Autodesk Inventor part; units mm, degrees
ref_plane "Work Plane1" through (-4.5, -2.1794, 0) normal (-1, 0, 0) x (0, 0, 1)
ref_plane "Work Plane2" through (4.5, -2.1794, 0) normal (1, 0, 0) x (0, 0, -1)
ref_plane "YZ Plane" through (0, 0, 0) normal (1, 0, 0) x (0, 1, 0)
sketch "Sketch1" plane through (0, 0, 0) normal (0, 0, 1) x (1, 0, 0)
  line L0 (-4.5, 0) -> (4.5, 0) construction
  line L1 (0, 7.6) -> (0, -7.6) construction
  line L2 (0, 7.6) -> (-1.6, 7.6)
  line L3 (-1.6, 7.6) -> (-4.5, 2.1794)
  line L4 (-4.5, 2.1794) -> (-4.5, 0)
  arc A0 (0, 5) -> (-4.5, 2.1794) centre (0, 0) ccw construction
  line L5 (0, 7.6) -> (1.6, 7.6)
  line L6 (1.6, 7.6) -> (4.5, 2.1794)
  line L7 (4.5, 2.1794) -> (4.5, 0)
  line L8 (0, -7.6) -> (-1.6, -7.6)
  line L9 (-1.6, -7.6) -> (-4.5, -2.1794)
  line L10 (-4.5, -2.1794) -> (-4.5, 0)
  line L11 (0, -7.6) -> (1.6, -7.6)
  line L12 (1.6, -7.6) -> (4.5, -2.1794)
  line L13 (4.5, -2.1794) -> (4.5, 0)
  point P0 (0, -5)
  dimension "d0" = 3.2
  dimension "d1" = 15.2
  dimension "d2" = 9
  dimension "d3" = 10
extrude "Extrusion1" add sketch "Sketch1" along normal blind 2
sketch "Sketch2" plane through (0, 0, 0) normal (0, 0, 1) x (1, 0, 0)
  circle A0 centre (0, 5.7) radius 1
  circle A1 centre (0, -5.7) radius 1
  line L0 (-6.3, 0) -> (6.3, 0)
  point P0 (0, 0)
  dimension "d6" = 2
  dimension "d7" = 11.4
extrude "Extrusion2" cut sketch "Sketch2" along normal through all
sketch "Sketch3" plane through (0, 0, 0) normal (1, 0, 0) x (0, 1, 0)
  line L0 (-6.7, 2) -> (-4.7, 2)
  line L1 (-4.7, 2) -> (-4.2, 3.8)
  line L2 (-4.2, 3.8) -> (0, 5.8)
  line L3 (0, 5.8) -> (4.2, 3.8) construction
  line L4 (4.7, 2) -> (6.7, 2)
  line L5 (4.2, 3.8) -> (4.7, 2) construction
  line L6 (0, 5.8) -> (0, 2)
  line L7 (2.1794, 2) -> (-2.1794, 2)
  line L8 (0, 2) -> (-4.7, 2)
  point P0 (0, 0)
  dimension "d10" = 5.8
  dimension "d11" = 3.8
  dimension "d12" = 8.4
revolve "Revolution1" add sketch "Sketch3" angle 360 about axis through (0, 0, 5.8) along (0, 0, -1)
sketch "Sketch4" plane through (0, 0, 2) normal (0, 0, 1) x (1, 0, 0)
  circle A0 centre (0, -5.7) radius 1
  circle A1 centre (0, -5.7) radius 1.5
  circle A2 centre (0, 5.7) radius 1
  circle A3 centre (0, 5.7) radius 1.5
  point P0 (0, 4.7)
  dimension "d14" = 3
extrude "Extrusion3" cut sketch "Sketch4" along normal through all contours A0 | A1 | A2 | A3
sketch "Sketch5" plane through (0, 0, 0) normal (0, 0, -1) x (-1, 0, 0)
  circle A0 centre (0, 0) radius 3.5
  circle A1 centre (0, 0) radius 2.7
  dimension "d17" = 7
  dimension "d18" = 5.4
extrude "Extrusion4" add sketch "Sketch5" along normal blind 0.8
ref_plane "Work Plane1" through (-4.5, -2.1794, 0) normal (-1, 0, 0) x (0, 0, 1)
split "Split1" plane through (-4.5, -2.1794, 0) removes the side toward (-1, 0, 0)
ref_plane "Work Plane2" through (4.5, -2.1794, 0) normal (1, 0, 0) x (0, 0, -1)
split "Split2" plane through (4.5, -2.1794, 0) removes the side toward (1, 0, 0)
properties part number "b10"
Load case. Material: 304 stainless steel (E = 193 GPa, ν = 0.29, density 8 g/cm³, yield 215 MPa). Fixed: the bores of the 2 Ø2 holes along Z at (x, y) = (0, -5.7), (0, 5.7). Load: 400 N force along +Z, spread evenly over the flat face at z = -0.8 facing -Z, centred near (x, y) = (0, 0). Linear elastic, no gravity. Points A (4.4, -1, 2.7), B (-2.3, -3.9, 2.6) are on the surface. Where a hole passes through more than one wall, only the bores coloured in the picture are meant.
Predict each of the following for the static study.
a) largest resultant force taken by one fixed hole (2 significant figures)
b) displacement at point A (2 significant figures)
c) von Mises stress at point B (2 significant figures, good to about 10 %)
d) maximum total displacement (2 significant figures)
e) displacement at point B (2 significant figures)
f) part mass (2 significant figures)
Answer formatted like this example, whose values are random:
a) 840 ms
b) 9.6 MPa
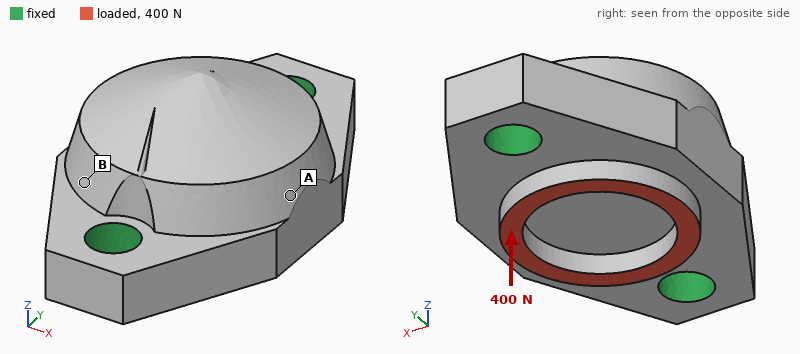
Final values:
a) 210 N
b) 1.1 µm
c) 21 MPa
d) 1.3 µm
e) 0.67 µm
f) 2.9 g
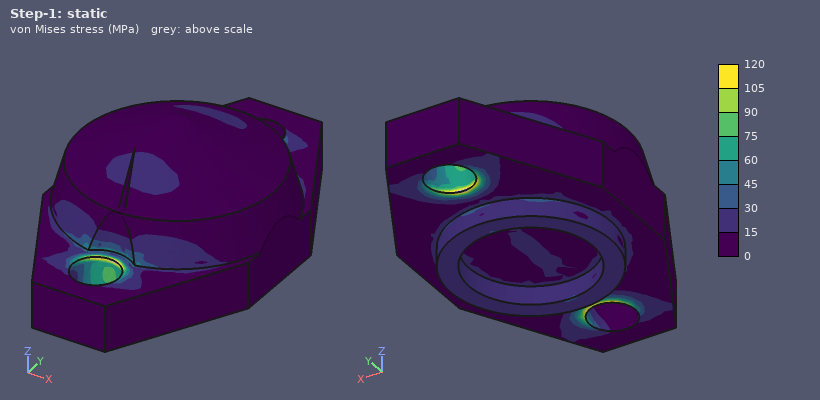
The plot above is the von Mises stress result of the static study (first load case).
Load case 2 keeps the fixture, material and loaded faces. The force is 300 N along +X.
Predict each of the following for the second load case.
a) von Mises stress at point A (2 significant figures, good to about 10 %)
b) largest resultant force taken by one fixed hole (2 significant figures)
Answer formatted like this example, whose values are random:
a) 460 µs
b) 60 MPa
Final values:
a) 11 MPa
b) 150 N
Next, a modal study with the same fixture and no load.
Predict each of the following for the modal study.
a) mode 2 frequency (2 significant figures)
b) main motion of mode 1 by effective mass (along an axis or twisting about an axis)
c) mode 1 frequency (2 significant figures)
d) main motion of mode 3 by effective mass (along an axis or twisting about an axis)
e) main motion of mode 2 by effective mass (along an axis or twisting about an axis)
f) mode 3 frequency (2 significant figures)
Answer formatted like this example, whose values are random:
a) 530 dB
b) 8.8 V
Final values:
a) 67 kHz
b) along X
c) 41 kHz
d) along X
e) along Z
f) 89 kHz
